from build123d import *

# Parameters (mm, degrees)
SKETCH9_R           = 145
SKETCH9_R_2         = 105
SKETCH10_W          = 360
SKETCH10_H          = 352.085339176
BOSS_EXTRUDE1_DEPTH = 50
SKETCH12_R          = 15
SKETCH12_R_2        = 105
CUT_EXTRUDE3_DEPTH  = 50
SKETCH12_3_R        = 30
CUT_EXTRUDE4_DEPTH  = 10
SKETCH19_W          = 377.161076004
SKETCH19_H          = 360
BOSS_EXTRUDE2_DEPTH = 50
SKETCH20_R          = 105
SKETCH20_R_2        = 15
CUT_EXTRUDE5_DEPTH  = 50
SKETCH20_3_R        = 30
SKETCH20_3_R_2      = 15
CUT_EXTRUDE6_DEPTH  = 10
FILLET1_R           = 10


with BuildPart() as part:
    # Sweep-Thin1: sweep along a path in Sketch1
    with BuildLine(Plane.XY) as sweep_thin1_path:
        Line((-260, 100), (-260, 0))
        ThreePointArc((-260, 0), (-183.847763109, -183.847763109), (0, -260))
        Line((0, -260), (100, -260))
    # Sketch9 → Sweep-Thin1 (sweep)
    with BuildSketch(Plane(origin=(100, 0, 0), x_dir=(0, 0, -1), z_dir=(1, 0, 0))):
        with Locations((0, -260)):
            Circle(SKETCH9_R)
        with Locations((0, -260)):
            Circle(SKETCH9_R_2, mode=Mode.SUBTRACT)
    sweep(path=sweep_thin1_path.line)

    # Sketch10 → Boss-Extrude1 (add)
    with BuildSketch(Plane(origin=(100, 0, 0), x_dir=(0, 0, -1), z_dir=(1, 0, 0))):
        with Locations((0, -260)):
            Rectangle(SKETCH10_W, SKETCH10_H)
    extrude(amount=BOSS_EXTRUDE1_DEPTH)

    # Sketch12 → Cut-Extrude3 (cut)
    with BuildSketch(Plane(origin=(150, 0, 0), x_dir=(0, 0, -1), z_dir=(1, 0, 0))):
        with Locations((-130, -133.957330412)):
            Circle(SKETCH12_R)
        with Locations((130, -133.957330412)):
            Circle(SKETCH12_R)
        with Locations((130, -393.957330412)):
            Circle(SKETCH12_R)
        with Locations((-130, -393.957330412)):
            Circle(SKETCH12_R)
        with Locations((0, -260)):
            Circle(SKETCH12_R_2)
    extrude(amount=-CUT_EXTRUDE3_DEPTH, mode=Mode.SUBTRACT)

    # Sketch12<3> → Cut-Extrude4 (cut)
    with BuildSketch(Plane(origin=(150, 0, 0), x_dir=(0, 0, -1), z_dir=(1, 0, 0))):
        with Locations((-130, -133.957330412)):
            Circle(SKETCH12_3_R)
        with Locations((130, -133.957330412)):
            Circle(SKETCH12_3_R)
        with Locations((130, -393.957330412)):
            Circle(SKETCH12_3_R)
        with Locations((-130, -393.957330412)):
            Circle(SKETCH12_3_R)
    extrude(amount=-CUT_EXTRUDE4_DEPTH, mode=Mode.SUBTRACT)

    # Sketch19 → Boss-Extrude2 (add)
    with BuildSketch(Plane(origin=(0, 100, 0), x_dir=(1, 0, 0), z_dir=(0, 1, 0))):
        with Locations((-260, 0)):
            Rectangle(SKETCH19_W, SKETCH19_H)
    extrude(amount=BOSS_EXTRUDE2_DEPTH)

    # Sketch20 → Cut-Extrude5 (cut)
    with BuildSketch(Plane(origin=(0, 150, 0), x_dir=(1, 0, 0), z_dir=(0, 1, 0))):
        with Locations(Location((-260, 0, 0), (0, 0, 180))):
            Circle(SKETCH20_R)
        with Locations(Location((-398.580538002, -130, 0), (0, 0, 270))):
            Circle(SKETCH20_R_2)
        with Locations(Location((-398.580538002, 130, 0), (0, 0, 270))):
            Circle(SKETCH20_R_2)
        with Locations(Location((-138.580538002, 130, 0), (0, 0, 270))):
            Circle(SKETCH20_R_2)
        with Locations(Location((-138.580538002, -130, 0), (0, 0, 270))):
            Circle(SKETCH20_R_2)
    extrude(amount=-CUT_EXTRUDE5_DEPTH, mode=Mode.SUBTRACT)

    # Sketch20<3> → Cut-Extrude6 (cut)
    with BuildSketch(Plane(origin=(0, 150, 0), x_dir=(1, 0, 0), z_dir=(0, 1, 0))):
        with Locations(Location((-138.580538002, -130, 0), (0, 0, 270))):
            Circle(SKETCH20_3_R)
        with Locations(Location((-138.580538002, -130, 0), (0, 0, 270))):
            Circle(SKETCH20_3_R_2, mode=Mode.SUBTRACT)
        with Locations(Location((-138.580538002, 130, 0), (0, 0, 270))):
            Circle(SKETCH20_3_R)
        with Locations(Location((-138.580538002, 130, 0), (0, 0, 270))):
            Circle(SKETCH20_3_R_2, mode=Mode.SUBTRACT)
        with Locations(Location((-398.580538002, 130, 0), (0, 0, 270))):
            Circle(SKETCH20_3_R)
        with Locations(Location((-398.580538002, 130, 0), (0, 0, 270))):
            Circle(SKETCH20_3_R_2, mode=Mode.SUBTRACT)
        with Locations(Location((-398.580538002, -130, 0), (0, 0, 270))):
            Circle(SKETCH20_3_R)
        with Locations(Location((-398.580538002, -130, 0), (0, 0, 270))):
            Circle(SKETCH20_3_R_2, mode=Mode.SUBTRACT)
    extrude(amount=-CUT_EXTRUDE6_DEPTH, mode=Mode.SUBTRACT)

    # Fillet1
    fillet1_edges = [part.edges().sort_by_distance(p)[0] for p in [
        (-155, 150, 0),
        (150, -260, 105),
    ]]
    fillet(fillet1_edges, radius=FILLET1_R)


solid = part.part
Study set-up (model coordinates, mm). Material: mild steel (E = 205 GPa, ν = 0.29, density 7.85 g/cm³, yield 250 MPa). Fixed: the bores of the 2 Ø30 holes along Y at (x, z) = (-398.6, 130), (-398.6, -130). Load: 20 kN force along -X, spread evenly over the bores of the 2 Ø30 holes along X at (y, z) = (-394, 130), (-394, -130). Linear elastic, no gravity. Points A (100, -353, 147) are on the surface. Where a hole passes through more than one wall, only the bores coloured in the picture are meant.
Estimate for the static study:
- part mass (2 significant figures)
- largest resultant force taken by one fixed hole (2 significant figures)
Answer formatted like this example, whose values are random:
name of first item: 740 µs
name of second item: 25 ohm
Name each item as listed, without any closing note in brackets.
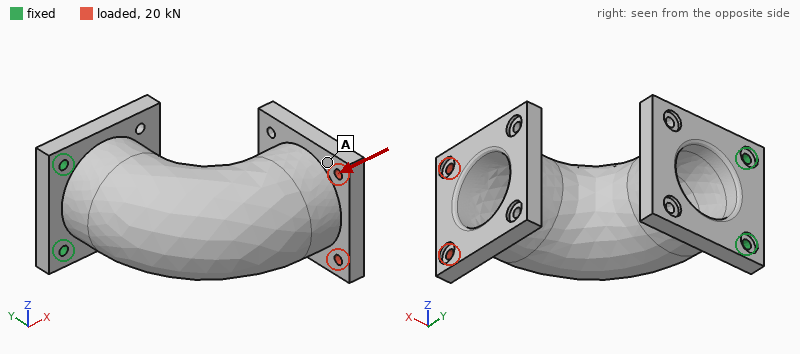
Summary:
part mass: 220 kg
largest resultant force taken by one fixed hole: 10 kN
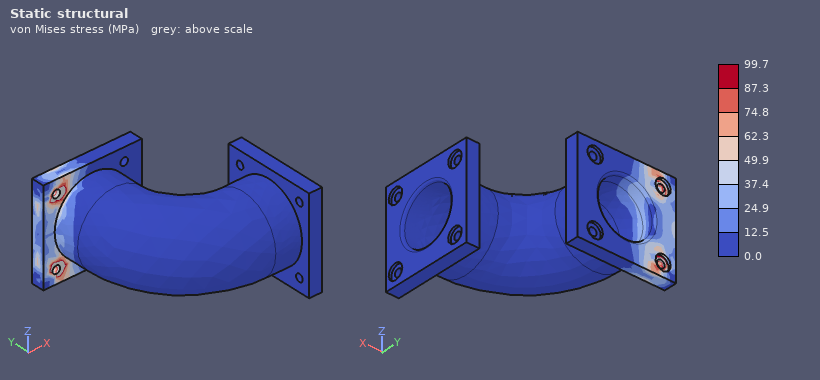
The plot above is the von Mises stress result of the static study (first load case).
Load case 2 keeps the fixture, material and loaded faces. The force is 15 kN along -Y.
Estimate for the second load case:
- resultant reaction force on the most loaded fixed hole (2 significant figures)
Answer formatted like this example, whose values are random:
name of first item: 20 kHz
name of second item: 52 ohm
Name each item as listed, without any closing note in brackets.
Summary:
resultant reaction force on the most loaded fixed hole: 7.5 kN
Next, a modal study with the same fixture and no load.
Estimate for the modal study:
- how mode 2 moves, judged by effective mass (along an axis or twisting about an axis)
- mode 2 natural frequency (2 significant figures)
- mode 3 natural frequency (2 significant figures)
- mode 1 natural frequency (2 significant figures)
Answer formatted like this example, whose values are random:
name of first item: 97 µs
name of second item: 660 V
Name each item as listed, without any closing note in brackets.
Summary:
how mode 2 moves, judged by effective mass: along Z
mode 2 natural frequency: 210 Hz
mode 3 natural frequency: 530 Hz
mode 1 natural frequency: 67 Hz
